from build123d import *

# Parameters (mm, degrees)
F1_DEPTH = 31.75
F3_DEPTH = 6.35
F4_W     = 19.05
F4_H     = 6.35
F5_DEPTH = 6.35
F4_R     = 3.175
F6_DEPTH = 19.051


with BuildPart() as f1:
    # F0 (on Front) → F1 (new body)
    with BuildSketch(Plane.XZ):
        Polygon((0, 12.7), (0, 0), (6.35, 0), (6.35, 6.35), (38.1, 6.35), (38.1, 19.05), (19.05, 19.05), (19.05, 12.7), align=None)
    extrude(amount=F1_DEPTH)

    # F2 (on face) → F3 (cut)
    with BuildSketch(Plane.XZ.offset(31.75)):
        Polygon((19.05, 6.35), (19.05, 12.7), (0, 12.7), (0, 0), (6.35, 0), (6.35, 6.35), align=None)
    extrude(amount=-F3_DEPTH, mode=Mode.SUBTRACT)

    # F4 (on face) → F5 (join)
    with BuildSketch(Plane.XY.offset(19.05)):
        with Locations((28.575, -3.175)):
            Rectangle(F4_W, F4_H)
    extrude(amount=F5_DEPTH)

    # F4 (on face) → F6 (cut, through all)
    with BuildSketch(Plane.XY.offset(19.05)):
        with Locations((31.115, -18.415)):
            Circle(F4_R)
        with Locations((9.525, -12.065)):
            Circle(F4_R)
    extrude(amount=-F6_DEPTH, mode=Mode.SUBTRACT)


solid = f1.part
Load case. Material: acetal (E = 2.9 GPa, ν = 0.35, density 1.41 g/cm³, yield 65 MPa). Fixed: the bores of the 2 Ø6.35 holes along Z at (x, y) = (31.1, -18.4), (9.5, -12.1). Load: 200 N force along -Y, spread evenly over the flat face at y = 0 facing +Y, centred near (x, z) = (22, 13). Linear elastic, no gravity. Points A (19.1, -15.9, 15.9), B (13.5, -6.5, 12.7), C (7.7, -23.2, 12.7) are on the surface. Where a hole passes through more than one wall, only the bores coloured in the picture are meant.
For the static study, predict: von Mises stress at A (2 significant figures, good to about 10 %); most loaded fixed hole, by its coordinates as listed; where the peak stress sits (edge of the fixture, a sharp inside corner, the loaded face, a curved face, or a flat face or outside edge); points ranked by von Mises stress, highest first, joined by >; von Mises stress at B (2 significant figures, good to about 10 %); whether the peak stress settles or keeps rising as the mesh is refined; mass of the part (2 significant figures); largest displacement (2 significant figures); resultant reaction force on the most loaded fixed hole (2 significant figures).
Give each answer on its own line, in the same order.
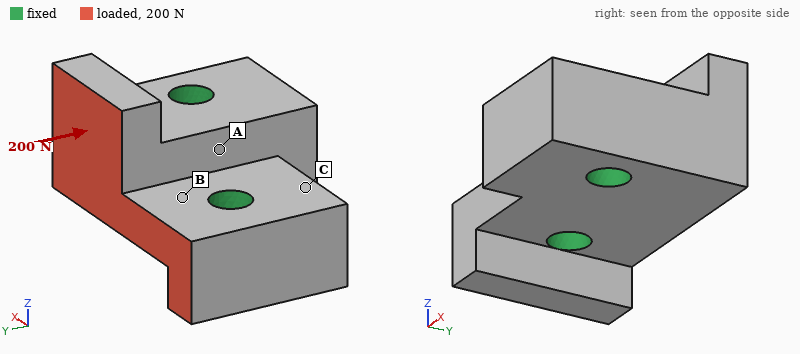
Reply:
0.53 MPa
(31.1, -18.4)
edge of the fixture
B > A > C
0.92 MPa
keeps rising
17 g
19 µm
130 N
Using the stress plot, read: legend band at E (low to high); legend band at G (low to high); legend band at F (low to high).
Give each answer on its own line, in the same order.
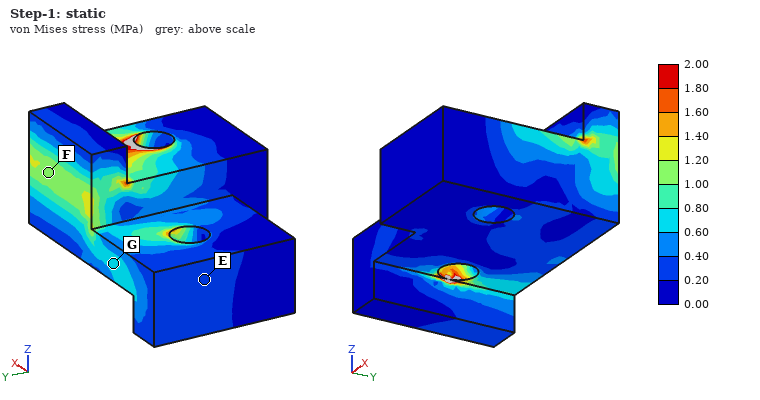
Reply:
0.20 to 0.40 MPa
0.60 to 0.80 MPa
1.00 to 1.20 MPa
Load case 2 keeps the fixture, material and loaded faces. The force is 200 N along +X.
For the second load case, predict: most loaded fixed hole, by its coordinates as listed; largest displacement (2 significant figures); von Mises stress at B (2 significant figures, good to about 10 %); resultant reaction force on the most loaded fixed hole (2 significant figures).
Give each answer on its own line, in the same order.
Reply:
(9.5, -12.1)
29 µm
2.2 MPa
160 N
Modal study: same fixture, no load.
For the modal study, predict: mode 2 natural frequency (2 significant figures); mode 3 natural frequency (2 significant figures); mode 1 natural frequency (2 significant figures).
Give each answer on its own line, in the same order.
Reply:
6900 Hz
7600 Hz
5800 Hz
